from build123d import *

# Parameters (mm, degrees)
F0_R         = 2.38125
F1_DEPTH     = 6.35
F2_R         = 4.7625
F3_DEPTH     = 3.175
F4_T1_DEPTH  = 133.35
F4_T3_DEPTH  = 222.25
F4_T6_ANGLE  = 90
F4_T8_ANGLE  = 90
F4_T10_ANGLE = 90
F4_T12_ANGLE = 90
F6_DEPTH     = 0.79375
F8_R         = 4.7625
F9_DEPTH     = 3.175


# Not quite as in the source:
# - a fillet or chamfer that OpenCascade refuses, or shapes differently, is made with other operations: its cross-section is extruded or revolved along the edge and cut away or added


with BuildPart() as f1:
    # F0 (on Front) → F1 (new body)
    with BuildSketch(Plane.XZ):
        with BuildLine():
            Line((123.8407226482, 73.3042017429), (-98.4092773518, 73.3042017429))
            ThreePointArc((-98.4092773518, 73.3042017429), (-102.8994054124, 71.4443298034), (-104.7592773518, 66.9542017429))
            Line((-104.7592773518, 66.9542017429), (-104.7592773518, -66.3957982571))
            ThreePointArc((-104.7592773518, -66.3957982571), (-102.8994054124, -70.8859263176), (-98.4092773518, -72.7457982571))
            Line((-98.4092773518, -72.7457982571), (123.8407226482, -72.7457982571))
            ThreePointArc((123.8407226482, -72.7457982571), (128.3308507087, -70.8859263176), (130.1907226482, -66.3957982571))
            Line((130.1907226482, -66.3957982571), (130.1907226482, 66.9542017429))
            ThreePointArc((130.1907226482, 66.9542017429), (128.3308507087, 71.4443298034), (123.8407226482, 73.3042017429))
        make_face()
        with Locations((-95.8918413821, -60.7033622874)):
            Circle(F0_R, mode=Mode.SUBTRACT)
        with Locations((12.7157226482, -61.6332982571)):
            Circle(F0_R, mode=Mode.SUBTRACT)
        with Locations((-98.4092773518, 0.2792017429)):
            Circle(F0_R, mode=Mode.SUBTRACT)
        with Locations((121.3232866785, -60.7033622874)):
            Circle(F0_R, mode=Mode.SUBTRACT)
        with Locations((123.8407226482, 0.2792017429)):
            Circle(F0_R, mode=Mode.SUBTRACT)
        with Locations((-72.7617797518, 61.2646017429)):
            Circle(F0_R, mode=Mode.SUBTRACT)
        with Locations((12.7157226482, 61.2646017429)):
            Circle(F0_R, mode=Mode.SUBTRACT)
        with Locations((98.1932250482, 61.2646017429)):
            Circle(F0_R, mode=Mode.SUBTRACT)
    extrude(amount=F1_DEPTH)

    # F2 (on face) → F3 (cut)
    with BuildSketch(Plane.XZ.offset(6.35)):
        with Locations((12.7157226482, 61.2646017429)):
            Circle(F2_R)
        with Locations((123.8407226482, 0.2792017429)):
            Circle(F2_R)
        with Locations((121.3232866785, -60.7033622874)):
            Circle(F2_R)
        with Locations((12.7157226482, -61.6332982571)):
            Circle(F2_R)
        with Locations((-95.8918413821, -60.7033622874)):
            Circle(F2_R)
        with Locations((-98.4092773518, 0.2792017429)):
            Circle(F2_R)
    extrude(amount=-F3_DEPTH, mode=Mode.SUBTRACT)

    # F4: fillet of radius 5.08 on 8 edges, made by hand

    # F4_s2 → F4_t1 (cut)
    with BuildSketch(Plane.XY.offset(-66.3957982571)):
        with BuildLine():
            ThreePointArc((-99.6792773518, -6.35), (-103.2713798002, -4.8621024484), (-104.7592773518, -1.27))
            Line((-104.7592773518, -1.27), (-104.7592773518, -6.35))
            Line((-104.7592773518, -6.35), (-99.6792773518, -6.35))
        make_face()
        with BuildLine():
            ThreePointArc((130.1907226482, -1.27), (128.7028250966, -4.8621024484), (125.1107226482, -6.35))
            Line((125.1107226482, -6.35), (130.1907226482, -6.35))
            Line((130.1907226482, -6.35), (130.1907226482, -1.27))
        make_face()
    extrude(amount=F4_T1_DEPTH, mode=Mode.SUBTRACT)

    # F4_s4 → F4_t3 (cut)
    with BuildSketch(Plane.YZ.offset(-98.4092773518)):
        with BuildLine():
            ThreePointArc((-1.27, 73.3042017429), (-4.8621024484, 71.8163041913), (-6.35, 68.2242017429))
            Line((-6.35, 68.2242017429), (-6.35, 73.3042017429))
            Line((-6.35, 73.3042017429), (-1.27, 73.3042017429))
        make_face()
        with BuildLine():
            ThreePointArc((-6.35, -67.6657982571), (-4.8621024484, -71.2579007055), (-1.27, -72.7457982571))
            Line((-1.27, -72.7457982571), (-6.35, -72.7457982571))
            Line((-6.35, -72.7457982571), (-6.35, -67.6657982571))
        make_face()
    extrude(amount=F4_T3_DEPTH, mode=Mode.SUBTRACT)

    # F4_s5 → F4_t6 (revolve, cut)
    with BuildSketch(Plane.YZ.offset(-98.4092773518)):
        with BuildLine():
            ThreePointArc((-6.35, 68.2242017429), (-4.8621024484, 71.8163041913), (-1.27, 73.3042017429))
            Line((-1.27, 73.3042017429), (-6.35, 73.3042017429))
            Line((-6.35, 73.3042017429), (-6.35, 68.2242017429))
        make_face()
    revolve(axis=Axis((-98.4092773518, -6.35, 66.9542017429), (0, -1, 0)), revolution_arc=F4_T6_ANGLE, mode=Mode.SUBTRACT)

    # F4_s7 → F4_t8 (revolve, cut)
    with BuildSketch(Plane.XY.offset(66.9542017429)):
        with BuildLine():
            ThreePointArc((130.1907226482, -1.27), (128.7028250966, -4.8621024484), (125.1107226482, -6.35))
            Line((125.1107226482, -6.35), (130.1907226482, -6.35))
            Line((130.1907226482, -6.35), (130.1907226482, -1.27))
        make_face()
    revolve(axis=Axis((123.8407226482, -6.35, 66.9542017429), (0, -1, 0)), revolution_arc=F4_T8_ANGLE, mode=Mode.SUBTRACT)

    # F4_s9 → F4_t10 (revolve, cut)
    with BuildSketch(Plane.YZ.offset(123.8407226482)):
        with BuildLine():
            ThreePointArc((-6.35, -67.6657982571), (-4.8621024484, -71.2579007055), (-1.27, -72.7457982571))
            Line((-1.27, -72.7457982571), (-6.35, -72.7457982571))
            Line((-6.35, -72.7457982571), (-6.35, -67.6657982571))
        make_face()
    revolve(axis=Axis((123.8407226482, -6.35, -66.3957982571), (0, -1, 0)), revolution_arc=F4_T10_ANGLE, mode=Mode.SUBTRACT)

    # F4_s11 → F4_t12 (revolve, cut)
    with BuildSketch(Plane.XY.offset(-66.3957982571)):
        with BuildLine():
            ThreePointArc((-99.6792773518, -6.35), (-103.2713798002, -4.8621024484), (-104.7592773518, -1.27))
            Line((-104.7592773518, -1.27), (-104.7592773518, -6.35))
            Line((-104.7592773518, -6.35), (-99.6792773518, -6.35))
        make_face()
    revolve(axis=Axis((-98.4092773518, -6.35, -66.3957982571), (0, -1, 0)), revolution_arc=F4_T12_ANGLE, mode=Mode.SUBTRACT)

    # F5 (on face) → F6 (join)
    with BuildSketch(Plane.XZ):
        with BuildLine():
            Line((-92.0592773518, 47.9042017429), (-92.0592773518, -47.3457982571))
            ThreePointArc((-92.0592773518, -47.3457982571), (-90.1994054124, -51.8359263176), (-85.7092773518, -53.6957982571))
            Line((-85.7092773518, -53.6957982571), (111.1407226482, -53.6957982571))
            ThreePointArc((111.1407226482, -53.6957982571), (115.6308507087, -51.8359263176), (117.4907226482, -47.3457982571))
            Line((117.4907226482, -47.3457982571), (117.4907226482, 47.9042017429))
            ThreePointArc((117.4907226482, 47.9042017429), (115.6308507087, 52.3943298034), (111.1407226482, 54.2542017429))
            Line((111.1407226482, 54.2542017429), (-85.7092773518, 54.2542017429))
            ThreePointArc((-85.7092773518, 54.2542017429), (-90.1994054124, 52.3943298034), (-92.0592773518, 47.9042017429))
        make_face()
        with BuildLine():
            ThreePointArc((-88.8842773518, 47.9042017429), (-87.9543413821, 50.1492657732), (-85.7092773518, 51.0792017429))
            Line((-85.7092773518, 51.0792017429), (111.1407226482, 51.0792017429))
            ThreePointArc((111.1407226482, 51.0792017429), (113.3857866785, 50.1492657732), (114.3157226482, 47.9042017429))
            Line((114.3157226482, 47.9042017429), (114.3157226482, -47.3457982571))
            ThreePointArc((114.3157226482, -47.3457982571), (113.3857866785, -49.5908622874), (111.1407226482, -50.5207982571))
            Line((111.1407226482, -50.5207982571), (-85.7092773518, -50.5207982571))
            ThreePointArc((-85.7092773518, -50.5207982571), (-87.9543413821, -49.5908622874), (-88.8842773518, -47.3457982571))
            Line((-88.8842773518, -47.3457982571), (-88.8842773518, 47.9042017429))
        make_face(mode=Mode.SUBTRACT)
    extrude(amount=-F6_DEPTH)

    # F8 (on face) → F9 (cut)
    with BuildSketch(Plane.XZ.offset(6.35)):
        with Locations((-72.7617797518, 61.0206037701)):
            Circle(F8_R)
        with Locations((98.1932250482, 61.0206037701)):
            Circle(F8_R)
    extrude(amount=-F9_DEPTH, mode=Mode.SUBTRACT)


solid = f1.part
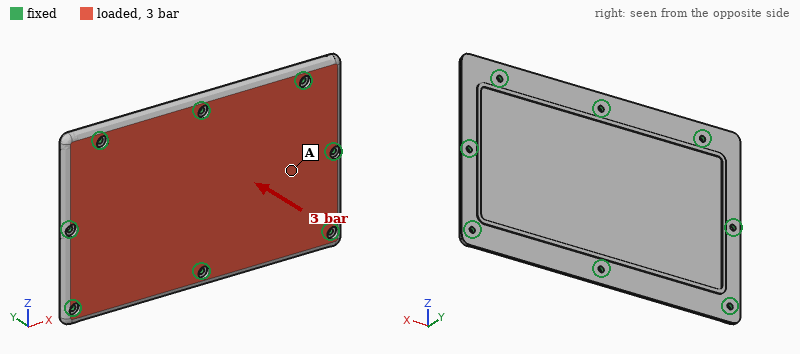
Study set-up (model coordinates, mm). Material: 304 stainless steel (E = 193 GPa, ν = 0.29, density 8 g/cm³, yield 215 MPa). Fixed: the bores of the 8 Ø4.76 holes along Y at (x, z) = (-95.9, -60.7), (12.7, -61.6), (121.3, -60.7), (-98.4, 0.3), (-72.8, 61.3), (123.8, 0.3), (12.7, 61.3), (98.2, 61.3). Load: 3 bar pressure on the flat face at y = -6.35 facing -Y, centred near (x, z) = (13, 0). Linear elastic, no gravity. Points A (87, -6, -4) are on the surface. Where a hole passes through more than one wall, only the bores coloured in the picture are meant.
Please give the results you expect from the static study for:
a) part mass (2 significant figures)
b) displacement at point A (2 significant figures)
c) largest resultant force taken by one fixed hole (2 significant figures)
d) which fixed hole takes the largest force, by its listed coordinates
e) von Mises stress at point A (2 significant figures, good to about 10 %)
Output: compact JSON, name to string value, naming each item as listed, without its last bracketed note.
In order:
{"part mass": "1.7 kg", "displacement at point A": "61 µm", "largest resultant force taken by one fixed hole": "3.4 kN", "which fixed hole takes the largest force, by its listed coordinates": "(12.7, -61.6)", "von Mises stress at point A": "24 MPa"}
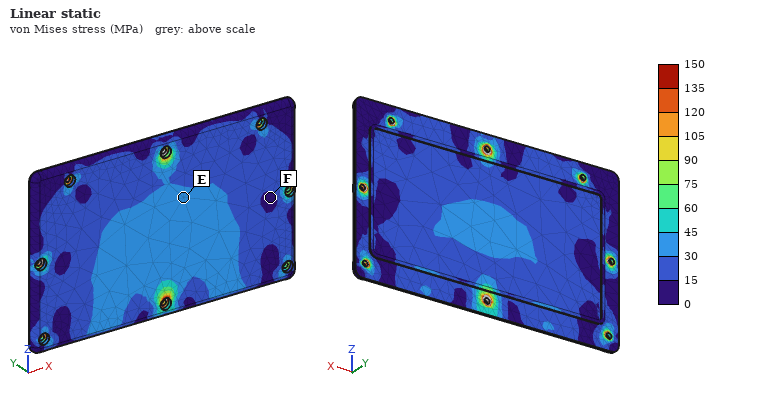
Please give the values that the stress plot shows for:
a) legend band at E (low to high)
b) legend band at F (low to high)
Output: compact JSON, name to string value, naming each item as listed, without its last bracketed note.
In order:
{"legend band at E": "30 to 45 MPa", "legend band at F": "0 to 15 MPa"}
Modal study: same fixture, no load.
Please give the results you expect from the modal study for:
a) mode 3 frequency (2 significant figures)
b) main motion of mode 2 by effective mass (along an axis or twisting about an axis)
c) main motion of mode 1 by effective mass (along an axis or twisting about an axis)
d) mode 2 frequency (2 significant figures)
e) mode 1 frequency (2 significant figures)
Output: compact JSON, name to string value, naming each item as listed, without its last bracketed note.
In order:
{"mode 3 frequency": "2700 Hz", "main motion of mode 2 by effective mass": "twisting about Z", "main motion of mode 1 by effective mass": "along Y", "mode 2 frequency": "1800 Hz", "mode 1 frequency": "1500 Hz"}
